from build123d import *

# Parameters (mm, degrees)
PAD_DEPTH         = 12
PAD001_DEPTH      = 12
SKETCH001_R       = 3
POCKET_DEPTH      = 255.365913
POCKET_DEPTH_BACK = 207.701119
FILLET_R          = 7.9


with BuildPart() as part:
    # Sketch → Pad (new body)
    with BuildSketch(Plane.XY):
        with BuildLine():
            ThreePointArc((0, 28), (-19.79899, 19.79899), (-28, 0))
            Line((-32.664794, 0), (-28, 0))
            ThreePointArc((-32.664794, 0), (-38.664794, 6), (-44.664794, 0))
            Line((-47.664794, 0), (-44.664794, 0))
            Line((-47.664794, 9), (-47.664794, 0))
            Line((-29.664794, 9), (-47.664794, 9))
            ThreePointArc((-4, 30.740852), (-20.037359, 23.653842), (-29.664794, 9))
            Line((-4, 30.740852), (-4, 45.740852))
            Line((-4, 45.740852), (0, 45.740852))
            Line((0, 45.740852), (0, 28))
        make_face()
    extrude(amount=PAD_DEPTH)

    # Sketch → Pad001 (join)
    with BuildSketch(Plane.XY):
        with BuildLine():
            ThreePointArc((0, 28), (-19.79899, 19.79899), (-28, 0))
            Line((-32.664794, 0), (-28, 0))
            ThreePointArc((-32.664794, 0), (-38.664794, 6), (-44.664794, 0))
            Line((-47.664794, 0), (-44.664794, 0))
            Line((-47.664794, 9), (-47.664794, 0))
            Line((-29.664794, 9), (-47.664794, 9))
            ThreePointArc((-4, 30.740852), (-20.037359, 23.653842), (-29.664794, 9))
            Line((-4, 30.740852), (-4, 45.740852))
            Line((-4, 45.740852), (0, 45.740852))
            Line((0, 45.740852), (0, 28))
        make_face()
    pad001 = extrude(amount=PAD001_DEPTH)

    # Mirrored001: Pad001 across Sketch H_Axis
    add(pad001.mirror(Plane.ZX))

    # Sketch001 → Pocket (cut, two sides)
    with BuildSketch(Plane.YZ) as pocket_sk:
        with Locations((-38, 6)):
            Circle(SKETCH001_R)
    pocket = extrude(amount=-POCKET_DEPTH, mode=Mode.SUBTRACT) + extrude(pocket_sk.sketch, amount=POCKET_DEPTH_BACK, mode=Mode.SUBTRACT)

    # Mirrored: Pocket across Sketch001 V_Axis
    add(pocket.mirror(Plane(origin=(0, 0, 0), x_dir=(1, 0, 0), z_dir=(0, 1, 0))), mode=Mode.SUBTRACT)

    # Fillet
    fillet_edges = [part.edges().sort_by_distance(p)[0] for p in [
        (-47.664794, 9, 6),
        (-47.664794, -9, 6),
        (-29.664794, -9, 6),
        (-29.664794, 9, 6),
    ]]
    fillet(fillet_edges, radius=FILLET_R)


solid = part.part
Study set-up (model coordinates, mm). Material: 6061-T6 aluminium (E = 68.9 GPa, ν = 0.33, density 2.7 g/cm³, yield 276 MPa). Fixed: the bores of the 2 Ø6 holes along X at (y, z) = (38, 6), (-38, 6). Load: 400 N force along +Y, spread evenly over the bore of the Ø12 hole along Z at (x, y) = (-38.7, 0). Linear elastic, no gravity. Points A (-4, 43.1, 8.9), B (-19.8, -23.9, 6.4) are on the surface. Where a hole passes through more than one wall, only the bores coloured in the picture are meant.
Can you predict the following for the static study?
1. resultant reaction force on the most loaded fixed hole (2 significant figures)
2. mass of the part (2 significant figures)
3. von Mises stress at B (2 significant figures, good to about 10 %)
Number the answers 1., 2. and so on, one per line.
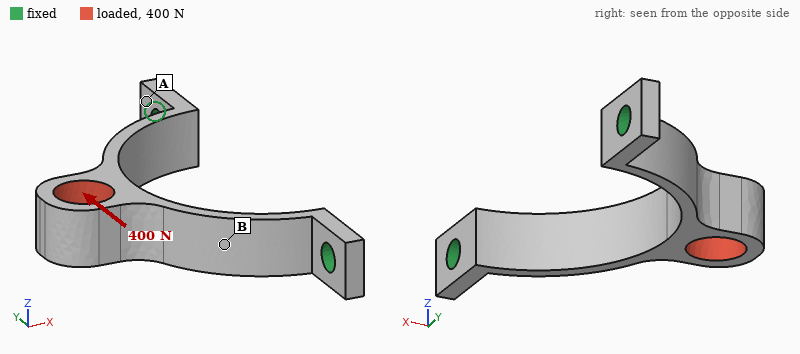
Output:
1. 280 N
2. 18 g
3. 22 MPa
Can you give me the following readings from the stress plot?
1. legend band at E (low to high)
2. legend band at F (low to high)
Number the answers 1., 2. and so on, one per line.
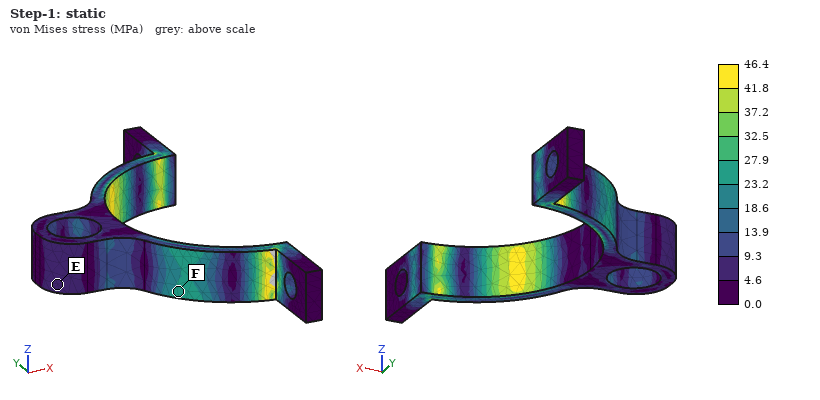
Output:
1. 4.6 to 9.3 MPa
2. 23.2 to 27.9 MPa
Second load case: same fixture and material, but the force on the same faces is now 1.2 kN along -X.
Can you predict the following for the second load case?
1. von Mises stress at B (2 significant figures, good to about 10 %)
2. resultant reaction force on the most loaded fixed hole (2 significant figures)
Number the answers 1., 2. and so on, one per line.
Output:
1. 42 MPa
2. 760 N
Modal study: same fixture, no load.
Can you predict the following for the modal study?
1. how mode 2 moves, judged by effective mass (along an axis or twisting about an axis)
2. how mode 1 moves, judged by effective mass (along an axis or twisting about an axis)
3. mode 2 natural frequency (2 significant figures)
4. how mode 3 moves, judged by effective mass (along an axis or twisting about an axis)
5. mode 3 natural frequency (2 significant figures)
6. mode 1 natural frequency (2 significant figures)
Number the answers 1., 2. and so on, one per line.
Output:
1. along Y
2. along Z
3. 3200 Hz
4. along X
5. 7200 Hz
6. 1700 Hz
